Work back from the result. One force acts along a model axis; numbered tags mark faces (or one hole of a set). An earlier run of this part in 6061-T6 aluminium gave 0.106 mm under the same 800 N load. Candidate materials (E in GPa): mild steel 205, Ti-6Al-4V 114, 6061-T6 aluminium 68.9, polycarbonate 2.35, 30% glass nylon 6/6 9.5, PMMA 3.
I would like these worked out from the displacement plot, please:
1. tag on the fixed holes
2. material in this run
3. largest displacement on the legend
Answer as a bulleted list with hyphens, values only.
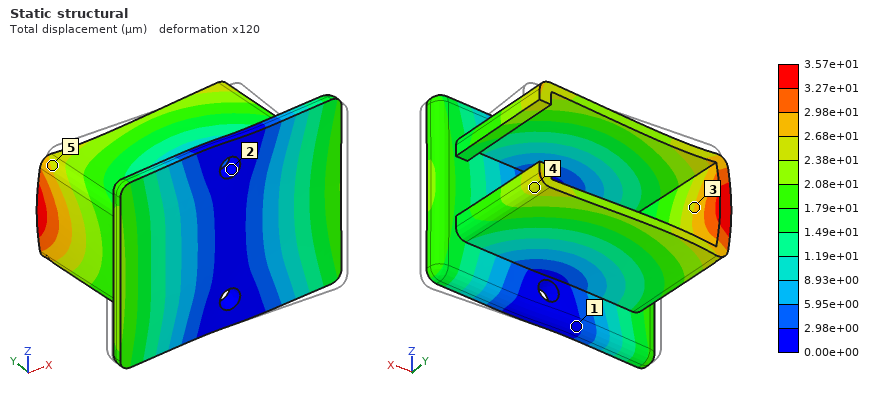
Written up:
- 2
- mild steel
- 3.57e+01 µm
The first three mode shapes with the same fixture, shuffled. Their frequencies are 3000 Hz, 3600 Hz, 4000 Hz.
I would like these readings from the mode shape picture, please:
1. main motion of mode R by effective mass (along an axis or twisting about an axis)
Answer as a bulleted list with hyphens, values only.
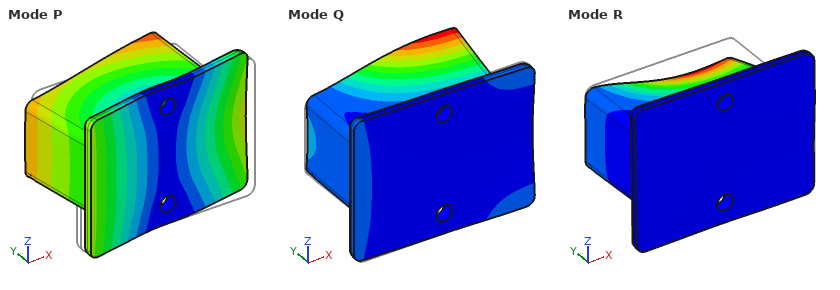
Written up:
- along Z
